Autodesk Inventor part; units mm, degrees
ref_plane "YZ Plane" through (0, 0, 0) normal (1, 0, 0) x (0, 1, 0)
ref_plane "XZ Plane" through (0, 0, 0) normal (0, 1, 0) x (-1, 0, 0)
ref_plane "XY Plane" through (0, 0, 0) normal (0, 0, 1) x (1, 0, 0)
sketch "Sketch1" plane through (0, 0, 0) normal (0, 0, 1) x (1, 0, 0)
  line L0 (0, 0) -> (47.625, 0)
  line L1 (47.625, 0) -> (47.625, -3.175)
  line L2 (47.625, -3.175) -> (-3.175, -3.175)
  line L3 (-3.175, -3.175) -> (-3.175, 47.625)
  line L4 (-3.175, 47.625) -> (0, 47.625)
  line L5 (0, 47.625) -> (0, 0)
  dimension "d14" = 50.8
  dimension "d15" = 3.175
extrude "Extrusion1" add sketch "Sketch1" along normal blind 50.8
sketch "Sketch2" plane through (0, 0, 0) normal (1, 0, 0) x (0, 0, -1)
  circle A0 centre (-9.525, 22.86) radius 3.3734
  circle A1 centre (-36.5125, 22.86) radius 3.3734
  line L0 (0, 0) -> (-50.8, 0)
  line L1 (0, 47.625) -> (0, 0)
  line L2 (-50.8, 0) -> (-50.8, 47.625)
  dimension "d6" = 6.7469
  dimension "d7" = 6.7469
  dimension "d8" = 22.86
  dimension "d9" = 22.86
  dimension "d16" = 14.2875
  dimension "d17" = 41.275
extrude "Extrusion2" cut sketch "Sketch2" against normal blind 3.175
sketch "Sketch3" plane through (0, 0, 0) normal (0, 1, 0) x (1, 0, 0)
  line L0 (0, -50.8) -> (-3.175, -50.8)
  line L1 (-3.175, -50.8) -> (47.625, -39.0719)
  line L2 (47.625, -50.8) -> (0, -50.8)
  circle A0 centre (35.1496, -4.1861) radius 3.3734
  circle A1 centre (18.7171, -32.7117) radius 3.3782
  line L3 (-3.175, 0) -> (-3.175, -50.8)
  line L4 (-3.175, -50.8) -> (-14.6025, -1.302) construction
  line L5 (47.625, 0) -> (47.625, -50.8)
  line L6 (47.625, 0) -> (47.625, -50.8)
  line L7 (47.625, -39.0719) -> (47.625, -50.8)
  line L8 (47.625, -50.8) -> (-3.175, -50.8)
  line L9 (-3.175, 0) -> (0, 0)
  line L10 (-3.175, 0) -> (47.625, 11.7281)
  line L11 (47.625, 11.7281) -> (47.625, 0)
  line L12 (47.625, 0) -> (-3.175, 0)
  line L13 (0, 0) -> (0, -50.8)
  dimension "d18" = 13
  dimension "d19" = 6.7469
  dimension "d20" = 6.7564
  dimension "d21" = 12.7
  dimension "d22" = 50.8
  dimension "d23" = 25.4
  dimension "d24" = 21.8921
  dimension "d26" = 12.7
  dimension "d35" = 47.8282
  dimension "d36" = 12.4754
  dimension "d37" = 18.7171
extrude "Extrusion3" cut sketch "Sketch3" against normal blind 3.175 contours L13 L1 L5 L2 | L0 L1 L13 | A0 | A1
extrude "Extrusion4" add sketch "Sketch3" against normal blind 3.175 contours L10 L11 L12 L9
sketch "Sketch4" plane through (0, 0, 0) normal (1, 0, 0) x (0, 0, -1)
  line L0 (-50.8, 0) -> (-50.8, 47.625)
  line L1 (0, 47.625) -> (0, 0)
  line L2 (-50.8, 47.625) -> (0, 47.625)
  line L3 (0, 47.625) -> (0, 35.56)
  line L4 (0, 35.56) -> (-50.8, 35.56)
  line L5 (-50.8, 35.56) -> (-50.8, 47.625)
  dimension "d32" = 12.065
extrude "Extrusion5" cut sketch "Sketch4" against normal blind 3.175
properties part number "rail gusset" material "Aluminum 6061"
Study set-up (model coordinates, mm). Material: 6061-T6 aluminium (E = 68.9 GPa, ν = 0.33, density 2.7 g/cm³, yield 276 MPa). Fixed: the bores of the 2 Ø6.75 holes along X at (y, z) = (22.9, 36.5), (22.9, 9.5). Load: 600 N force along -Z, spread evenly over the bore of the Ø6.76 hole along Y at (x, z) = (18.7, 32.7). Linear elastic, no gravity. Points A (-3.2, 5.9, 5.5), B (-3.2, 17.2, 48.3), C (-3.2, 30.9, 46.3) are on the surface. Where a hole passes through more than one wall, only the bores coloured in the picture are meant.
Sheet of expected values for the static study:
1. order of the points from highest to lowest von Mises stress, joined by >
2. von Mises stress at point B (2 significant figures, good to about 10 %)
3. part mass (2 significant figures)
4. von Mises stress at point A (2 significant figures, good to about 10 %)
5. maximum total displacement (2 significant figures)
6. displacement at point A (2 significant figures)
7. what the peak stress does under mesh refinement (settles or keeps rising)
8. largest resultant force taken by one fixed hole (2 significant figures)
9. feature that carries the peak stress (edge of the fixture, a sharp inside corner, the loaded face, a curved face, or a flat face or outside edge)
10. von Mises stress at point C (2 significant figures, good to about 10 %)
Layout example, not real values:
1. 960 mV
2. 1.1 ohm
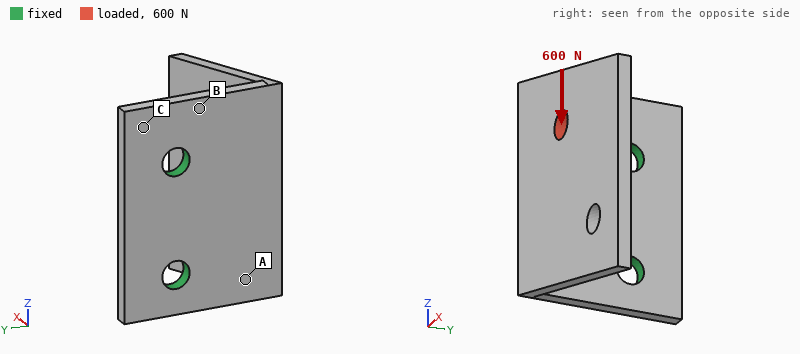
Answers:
1. B > A > C
2. 67 MPa
3. 36 g
4. 49 MPa
5. 0.51 mm
6. 0.092 mm
7. keeps rising
8. 650 N
9. edge of the fixture
10. 17 MPa
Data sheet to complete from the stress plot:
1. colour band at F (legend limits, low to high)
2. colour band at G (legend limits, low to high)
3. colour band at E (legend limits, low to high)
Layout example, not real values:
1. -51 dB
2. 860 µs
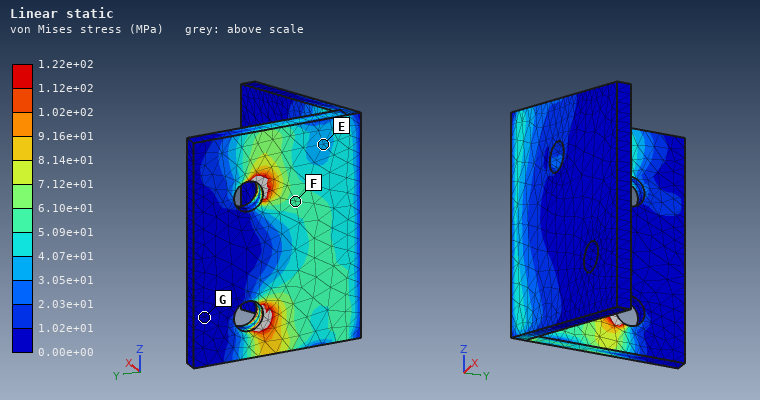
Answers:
1. 5.09e+01 to 6.10e+01 MPa
2. 0.00e+00 to 1.02e+01 MPa
3. 3.05e+01 to 4.07e+01 MPa
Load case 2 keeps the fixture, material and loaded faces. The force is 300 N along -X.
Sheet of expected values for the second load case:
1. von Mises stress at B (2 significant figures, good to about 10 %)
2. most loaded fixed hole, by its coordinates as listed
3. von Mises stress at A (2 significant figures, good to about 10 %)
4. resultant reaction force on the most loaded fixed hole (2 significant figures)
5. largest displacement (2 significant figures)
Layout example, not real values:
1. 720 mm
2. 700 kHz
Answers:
1. 57 MPa
2. (22.9, 36.5)
3. 27 MPa
4. 230 N
5. 0.44 mm
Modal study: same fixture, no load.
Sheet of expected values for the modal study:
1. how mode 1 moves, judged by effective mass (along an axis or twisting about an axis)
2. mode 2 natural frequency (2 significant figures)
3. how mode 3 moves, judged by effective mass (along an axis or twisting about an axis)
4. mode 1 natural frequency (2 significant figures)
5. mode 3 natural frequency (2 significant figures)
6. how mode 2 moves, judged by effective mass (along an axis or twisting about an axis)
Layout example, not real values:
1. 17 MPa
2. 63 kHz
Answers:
1. along Y
2. 1300 Hz
3. along X
4. 630 Hz
5. 2100 Hz
6. along Z
